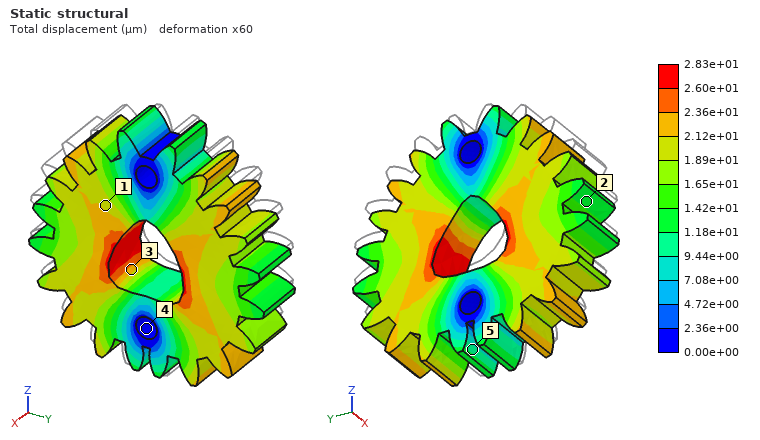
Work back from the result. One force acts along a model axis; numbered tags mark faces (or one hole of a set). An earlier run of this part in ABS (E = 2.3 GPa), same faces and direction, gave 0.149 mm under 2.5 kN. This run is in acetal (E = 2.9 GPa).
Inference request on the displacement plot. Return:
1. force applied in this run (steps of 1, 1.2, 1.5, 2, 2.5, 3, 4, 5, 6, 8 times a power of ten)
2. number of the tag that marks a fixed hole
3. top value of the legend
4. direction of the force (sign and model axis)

600 N
4
2.83e+01 µm
-Z
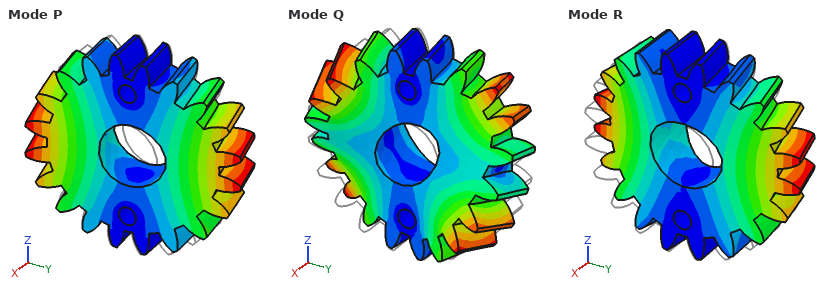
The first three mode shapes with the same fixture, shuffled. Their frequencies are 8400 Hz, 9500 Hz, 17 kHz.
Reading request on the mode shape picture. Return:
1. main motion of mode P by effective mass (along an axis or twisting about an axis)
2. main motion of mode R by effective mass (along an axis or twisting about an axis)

twisting about Z
along X
